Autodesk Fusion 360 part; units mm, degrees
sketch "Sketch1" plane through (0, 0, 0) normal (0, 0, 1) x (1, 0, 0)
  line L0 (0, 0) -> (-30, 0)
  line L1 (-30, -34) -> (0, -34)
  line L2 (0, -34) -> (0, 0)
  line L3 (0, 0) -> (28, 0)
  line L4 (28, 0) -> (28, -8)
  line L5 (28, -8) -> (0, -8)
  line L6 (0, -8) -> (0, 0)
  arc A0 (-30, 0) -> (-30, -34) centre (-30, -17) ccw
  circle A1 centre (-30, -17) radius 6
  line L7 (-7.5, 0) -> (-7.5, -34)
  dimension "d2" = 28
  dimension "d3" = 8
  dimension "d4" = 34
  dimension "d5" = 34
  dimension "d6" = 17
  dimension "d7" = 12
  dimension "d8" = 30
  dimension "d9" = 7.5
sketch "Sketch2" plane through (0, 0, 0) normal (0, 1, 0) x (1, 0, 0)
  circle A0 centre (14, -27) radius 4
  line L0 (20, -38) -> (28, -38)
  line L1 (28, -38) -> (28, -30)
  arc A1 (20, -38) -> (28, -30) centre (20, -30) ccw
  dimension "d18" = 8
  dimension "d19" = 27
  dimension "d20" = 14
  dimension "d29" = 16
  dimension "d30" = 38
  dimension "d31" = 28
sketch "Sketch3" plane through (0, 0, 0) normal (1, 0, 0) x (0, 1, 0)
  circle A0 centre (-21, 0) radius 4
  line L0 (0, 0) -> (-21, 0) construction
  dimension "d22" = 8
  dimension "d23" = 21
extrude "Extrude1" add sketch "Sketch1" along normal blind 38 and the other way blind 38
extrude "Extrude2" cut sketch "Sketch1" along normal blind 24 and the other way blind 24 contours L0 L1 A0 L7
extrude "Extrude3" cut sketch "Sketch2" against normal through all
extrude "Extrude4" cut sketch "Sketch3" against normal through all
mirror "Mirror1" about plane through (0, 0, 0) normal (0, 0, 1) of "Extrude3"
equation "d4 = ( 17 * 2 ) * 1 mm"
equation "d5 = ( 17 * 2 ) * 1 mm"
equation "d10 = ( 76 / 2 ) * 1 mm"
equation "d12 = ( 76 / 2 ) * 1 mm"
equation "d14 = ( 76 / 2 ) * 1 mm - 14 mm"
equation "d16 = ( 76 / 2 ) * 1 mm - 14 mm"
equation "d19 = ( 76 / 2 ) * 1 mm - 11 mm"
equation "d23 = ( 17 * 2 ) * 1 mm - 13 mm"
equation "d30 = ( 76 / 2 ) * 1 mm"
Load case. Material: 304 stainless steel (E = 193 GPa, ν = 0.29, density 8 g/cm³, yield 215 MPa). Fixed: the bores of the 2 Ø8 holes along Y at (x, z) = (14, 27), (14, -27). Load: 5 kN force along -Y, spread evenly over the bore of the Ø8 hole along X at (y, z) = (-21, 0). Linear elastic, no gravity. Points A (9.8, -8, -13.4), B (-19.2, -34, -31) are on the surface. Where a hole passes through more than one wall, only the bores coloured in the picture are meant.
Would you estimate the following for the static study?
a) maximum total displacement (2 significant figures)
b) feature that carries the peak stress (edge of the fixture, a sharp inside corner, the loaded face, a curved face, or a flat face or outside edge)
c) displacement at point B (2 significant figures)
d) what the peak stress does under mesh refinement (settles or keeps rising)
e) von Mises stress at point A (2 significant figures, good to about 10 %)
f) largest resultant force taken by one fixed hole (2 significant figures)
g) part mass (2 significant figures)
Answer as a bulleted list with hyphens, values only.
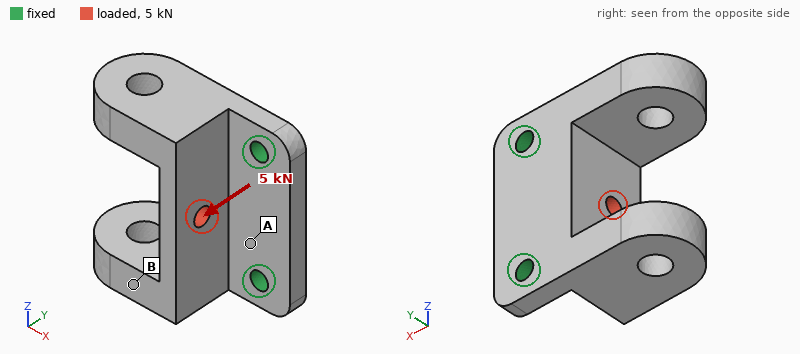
- 82 µm
- edge of the fixture
- 57 µm
- keeps rising
- 43 MPa
- 2.5 kN
- 530 g
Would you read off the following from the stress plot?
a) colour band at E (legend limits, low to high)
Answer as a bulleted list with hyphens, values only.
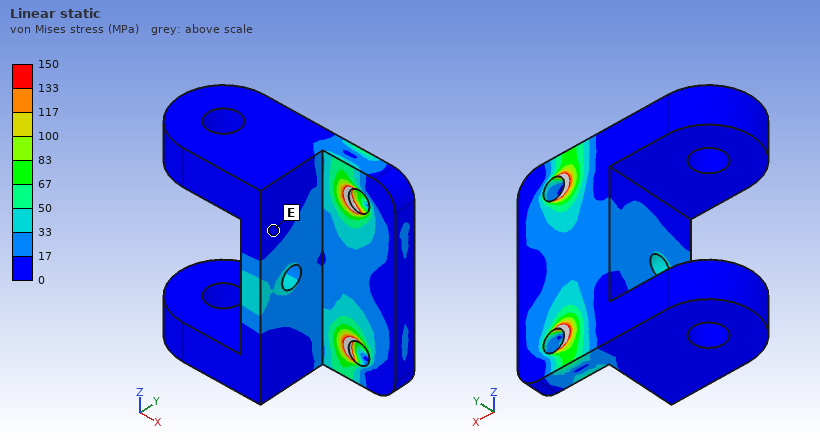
- 0 to 17 MPa
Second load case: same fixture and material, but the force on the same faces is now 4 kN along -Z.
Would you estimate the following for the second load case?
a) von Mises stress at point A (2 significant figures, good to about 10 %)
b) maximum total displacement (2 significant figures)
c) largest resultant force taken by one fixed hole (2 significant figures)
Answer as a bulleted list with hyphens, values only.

- 20 MPa
- 20 µm
- 2.6 kN
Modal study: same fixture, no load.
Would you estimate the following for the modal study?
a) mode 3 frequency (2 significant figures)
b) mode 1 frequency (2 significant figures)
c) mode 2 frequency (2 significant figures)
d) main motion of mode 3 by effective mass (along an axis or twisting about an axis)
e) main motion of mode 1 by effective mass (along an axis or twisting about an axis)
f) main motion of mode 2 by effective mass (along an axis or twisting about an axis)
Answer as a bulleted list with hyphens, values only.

- 3600 Hz
- 1400 Hz
- 2000 Hz
- along Z
- along Y
- twisting about X
